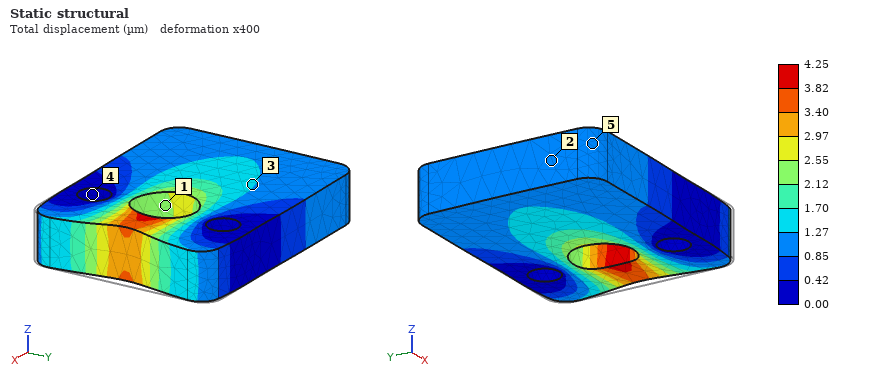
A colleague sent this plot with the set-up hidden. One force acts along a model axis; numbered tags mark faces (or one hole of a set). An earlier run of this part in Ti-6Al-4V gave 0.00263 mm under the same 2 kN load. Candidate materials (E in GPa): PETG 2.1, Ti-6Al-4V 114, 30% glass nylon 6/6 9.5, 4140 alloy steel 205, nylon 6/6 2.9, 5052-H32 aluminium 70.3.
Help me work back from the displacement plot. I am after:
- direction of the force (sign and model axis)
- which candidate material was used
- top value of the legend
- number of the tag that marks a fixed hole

-X
5052-H32 aluminium
4.25 µm
4
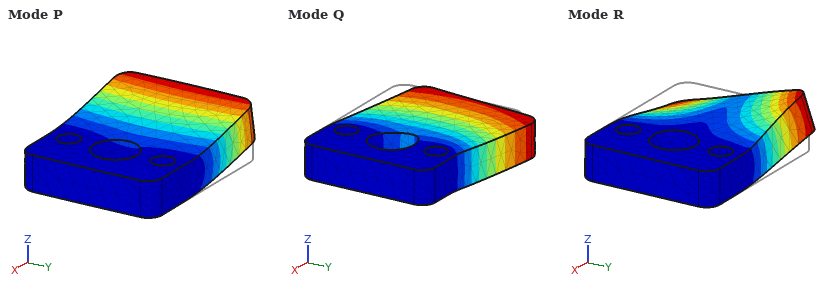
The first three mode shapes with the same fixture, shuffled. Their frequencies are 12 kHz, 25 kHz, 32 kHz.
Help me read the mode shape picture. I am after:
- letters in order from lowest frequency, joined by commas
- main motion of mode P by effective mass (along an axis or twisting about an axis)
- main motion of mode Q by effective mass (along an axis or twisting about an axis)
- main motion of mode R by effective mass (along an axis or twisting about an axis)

P, R, Q
along Z
along Y
twisting about X
